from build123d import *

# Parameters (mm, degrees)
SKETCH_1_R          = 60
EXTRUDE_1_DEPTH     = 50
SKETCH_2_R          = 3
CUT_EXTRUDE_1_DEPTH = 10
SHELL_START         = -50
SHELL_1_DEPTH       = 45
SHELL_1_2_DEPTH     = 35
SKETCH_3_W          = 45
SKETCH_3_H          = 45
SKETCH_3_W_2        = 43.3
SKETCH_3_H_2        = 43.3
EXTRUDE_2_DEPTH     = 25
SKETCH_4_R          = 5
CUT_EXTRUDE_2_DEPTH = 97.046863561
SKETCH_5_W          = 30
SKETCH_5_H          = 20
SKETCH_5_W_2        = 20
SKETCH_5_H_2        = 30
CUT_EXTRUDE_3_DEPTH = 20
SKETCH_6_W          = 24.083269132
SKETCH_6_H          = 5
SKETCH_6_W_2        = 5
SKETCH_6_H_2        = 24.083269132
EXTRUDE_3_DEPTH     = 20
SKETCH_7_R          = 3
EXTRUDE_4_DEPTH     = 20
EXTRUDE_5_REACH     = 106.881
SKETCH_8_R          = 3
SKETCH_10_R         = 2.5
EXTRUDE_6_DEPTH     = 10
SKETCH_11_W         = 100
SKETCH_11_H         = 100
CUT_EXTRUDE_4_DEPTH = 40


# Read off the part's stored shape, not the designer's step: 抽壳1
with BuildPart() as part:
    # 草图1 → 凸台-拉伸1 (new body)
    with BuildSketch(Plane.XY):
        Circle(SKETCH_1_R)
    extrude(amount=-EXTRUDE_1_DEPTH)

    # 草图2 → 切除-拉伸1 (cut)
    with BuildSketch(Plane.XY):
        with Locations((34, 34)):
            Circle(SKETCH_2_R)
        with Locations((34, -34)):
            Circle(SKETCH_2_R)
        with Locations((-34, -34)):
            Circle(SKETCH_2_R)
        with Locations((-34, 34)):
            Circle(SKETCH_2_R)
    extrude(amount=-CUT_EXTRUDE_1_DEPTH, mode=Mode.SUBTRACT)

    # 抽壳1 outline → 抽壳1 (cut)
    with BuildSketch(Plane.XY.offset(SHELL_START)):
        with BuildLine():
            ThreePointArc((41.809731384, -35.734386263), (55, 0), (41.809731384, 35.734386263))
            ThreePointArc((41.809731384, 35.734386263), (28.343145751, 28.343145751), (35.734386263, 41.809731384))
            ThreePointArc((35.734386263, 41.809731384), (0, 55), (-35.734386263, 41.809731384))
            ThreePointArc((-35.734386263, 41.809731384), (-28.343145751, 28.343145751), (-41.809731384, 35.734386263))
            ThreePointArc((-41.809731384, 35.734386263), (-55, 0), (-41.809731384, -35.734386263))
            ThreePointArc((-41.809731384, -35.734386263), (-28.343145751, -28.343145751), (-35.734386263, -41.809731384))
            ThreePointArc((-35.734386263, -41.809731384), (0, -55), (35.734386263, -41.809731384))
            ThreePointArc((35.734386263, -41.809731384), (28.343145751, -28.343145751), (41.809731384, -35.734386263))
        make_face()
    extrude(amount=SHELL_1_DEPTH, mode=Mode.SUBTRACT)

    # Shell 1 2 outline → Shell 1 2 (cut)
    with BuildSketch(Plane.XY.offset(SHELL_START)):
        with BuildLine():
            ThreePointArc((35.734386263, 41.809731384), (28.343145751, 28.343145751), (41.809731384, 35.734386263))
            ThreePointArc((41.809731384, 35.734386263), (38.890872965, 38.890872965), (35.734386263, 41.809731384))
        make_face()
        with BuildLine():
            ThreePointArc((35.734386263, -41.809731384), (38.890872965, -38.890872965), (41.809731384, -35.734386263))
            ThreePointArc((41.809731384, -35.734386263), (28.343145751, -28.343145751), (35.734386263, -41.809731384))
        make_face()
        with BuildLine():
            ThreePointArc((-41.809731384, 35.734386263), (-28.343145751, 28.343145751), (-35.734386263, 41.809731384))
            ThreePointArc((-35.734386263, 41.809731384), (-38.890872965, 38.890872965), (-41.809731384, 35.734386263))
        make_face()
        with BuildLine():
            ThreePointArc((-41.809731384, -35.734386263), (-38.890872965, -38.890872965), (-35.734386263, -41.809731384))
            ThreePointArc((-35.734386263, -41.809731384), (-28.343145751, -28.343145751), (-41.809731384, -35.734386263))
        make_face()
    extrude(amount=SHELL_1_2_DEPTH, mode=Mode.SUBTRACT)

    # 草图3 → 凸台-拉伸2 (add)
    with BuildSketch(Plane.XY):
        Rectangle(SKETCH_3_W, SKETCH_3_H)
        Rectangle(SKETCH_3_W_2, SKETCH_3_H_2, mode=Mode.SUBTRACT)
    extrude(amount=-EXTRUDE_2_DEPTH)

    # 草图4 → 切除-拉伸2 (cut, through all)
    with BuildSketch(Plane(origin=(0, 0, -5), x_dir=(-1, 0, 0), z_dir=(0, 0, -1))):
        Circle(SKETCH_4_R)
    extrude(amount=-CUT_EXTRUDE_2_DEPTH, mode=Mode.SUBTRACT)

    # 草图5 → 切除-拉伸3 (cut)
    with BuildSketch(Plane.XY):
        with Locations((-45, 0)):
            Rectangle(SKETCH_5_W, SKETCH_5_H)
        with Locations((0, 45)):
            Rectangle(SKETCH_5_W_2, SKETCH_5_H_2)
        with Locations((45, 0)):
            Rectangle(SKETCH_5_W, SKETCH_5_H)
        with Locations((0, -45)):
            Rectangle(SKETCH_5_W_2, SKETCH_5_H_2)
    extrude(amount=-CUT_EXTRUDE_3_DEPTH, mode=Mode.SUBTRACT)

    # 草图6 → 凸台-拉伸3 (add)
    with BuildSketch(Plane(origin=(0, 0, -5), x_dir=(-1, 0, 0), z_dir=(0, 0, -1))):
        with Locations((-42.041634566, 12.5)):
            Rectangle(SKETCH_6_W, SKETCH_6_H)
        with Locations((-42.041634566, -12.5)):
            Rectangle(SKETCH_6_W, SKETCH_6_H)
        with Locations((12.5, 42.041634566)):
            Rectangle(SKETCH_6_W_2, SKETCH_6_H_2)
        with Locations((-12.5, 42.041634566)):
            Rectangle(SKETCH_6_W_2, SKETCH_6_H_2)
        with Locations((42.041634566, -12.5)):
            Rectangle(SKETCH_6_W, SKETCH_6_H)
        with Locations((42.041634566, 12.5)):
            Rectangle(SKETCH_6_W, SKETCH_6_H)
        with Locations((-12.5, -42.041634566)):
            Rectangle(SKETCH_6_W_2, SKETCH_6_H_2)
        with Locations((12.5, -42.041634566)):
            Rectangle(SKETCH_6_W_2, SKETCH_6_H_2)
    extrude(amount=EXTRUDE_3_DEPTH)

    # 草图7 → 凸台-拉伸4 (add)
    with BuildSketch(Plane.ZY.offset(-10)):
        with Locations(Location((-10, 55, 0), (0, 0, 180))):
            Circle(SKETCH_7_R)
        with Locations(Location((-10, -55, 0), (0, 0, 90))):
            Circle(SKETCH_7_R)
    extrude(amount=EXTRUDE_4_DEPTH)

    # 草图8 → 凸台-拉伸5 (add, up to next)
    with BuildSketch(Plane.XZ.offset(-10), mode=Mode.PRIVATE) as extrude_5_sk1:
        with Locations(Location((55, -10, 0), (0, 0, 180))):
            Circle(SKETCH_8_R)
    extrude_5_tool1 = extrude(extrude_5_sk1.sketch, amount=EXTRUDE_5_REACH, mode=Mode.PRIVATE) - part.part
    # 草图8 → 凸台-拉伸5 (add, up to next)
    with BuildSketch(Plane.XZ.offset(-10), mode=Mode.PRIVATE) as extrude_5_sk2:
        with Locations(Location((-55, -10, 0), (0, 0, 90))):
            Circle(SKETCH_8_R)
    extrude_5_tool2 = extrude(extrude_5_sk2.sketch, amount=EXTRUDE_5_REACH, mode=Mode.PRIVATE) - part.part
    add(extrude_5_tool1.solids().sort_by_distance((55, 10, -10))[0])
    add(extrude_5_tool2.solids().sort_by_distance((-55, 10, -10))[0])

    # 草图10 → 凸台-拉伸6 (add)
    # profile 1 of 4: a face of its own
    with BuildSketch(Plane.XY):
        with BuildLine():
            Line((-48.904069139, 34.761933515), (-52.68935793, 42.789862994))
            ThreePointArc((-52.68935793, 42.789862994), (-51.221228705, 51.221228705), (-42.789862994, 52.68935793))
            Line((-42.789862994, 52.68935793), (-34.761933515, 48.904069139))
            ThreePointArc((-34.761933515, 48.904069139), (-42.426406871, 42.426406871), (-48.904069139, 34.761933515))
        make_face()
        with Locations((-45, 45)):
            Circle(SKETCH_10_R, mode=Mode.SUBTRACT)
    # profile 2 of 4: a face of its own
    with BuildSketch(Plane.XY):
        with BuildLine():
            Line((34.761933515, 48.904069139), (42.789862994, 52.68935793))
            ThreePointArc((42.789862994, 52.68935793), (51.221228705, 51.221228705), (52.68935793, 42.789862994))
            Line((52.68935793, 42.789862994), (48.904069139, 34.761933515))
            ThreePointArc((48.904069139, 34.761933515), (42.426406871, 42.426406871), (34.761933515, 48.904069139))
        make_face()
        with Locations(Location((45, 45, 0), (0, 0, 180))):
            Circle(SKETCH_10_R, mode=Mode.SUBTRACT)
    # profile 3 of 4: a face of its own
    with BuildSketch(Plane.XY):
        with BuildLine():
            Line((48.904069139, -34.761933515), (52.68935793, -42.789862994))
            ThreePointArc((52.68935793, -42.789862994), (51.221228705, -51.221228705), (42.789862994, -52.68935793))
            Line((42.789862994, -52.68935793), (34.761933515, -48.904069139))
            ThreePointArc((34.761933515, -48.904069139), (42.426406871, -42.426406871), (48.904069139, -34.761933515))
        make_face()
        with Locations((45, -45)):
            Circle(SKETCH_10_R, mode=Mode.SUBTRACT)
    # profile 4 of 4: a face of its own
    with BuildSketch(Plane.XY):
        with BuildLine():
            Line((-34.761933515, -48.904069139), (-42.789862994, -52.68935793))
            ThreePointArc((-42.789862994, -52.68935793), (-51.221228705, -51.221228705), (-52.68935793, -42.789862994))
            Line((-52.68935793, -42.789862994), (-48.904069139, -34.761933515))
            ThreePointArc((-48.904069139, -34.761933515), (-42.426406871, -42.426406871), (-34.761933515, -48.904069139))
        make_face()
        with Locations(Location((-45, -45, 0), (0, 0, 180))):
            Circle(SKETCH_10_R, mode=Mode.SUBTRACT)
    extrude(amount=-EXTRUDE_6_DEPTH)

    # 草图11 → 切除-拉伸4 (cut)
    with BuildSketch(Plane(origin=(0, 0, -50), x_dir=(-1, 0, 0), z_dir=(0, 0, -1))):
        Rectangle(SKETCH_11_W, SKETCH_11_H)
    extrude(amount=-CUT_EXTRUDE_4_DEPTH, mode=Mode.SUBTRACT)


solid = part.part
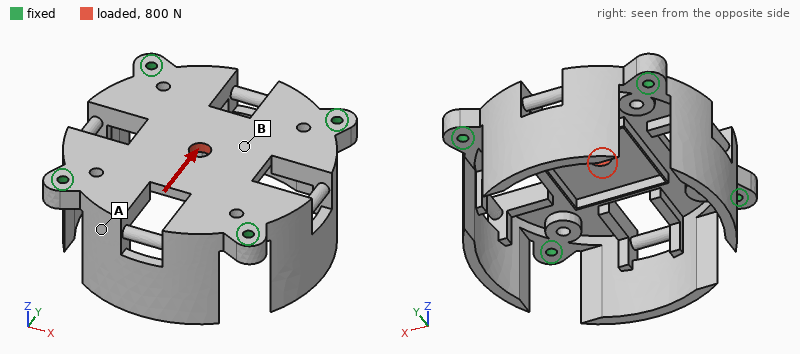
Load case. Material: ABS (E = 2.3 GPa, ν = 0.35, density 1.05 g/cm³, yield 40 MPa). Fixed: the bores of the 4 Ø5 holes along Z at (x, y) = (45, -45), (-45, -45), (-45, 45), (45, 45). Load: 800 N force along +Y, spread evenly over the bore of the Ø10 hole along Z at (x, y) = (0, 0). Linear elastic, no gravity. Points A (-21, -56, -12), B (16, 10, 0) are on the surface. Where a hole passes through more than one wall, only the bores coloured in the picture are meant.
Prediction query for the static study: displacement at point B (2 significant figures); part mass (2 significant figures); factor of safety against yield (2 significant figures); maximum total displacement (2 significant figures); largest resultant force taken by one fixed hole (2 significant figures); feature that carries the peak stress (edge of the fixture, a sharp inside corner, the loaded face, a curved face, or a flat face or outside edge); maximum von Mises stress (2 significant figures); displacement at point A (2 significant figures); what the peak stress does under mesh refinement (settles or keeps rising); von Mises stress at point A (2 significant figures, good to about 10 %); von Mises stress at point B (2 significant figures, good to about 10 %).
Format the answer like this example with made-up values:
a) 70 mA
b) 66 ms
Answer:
a) 45 µm
b) 120 g
c) 4.5
d) 82 µm
e) 240 N
f) the loaded face
g) 8.9 MPa
h) 29 µm
i) settles
j) 0.71 MPa
k) 2.0 MPa
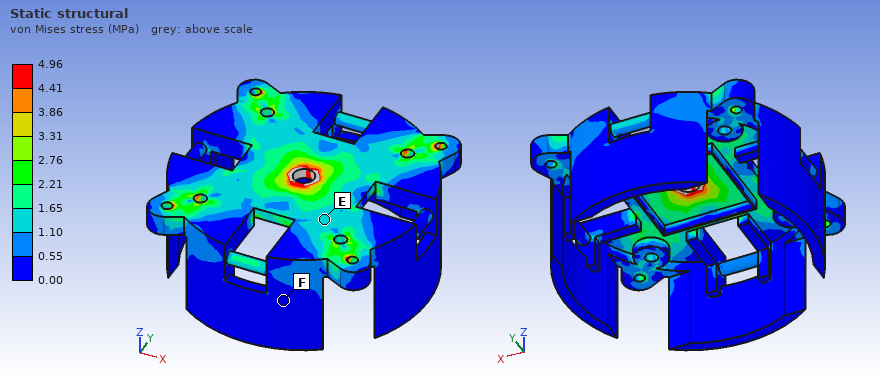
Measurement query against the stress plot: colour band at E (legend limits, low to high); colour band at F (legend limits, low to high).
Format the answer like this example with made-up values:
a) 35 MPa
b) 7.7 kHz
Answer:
a) 1.10 to 1.65 MPa
b) 0.00 to 0.55 MPa
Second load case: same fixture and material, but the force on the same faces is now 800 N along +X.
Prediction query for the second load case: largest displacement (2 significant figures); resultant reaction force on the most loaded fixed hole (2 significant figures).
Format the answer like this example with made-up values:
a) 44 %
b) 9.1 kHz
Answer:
a) 82 µm
b) 240 N
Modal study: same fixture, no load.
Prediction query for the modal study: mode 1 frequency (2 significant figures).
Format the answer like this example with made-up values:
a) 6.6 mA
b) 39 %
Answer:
a) 450 Hz
